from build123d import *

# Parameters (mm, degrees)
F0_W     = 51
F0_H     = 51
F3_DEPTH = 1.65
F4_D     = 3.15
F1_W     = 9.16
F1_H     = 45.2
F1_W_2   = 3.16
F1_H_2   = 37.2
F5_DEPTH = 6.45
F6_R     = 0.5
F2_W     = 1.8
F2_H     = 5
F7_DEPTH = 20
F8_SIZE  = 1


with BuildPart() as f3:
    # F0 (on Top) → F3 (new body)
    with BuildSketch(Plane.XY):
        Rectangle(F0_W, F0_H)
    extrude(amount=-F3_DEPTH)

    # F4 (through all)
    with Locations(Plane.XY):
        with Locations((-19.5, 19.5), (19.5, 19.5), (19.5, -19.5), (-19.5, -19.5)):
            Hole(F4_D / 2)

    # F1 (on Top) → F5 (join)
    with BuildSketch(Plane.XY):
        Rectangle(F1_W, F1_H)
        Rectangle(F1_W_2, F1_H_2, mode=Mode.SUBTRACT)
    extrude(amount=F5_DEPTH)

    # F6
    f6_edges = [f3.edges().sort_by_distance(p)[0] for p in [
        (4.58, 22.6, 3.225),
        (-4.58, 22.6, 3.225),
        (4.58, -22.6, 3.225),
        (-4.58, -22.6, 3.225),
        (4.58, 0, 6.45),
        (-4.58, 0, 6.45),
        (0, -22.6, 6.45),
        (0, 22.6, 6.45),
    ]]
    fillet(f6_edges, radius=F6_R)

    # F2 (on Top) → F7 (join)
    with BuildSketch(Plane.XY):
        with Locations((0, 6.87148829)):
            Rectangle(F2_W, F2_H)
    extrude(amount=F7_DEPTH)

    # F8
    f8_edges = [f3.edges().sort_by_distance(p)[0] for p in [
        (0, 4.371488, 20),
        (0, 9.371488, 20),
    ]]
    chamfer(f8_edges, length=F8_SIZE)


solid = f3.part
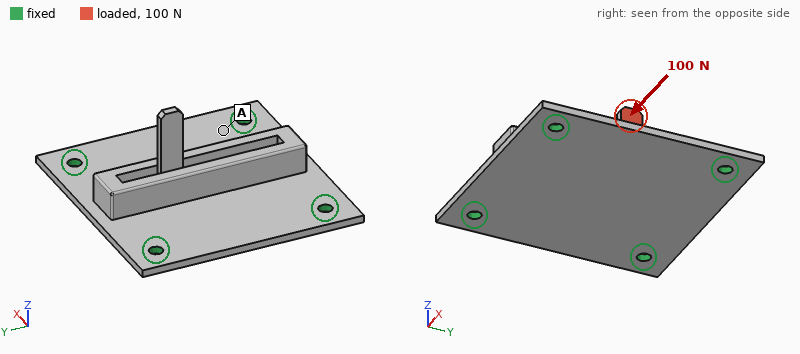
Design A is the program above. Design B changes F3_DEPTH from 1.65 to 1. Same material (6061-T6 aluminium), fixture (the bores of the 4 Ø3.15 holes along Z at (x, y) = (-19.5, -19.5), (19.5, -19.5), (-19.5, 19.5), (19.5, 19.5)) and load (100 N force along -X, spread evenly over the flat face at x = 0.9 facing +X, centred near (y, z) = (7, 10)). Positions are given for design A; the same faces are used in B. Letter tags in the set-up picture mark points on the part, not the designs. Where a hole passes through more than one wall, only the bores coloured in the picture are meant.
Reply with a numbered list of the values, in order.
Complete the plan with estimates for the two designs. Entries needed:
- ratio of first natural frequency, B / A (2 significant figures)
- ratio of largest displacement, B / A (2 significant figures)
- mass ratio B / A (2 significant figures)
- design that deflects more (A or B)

1. 0.62
2. 1.2
3. 0.74
4. B
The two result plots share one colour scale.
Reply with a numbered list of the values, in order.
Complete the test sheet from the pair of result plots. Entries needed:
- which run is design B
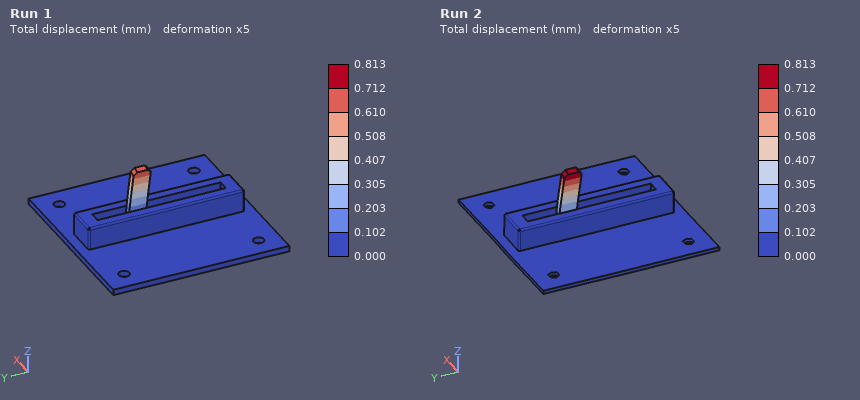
1. Run 2
